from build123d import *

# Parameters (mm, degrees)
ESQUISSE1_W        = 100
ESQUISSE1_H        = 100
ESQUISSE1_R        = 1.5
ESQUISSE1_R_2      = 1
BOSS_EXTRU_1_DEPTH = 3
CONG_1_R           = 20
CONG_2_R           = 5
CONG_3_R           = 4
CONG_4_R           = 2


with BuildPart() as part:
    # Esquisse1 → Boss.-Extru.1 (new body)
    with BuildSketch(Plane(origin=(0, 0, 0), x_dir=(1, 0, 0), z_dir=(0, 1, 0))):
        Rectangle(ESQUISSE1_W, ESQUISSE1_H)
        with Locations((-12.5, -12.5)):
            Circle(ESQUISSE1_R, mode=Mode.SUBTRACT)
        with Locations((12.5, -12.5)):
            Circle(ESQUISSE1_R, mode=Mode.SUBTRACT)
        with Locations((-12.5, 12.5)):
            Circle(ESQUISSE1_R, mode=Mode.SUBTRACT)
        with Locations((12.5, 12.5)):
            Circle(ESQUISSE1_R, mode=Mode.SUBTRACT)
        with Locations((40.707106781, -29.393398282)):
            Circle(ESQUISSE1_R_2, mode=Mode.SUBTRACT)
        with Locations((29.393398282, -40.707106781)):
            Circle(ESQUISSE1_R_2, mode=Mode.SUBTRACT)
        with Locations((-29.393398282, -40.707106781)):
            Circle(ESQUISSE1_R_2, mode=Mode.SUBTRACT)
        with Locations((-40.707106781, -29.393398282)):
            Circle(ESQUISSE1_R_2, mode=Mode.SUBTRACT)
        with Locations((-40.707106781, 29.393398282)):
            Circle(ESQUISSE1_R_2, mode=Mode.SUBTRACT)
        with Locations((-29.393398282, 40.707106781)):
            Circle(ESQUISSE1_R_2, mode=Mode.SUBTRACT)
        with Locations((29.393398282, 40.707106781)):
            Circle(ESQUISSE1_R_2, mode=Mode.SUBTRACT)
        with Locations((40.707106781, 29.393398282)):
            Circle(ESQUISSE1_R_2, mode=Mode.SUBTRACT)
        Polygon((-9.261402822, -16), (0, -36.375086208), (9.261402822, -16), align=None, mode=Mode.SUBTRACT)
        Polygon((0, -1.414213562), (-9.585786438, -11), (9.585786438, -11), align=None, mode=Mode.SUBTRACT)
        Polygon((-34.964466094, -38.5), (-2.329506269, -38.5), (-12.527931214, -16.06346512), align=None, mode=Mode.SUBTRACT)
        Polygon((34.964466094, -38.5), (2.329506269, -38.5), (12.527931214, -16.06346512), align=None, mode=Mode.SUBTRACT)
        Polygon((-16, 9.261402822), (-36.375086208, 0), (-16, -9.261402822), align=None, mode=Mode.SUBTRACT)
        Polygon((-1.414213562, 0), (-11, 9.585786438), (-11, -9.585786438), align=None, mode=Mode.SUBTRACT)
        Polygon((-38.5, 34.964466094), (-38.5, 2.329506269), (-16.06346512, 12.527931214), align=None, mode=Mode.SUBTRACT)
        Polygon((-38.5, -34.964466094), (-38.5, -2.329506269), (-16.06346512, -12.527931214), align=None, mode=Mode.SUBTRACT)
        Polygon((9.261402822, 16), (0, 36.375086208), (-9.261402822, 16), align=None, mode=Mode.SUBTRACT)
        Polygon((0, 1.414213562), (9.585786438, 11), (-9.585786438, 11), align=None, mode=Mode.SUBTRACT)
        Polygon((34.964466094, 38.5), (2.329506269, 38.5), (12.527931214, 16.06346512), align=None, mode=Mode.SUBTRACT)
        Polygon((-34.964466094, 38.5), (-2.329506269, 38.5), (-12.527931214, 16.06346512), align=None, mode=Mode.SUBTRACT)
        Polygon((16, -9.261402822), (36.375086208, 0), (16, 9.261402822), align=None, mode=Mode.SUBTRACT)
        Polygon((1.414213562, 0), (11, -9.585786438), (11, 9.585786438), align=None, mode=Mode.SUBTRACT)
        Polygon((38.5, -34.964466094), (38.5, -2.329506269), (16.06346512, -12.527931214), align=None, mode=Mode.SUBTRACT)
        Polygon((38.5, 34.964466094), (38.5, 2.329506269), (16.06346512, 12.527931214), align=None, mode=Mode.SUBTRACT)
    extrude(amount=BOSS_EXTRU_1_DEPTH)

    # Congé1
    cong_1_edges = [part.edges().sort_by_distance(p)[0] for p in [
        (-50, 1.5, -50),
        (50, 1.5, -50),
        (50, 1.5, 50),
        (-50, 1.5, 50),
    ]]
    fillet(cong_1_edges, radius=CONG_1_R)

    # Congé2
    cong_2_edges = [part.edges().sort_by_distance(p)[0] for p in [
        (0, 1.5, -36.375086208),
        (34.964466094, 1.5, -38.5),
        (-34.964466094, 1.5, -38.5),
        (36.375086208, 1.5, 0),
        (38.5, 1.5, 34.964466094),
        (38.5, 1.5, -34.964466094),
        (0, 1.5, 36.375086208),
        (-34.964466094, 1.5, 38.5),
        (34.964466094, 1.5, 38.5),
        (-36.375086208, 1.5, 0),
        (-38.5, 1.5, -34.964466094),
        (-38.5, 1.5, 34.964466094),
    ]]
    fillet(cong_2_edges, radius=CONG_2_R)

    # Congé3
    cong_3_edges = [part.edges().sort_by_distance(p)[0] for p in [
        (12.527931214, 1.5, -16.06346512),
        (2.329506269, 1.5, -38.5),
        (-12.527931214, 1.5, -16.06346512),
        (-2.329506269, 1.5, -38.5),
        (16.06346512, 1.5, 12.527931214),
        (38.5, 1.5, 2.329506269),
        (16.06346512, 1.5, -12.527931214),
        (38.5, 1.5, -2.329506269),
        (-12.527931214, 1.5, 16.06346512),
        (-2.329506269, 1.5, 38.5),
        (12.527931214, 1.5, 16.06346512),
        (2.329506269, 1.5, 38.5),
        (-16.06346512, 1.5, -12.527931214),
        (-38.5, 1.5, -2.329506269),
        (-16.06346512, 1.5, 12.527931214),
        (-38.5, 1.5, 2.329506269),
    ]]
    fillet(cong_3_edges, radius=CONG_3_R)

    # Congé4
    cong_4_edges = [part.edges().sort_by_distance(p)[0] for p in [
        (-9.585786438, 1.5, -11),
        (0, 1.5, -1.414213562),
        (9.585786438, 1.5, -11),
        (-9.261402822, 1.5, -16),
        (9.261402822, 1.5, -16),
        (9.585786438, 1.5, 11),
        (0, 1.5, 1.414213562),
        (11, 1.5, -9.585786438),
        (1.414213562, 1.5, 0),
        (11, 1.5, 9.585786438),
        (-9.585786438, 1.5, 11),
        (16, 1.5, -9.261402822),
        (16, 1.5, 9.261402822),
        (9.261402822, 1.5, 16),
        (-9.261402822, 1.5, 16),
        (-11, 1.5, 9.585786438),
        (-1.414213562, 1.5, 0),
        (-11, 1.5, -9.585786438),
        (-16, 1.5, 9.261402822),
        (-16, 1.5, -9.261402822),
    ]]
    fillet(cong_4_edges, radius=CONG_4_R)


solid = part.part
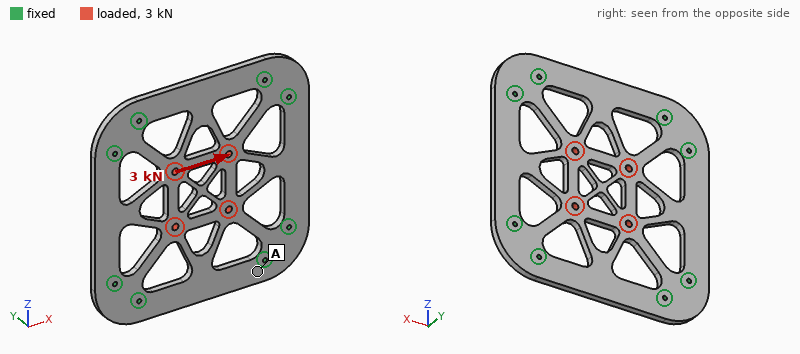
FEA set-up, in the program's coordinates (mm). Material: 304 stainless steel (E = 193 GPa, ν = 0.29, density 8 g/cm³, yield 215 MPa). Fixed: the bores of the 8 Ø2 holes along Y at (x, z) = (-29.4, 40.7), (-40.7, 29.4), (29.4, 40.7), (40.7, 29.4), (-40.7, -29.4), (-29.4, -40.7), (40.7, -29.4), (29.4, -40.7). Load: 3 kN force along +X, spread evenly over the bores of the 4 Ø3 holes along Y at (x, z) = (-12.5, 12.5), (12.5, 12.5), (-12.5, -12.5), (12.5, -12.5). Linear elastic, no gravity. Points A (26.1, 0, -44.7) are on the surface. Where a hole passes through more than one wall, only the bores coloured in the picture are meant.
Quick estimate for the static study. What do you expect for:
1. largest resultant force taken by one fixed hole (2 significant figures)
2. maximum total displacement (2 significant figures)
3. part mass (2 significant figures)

540 N
9.1 µm
150 g
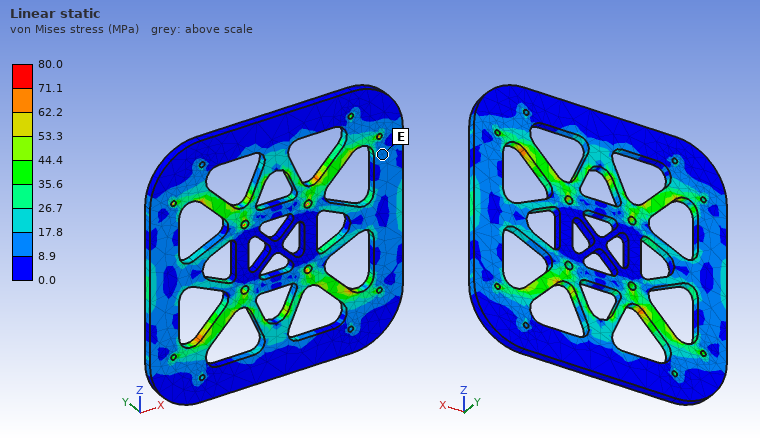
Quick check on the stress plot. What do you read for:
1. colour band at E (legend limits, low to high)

8.9 to 17.8 MPa
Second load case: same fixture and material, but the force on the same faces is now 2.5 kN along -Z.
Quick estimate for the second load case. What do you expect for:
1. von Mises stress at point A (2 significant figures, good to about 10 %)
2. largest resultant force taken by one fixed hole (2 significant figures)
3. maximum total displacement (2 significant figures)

6.1 MPa
450 N
7.6 µm
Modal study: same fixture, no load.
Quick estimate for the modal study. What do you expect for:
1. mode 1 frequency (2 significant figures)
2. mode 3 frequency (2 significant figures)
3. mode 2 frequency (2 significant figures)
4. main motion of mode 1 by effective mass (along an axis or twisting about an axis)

2000 Hz
3600 Hz
3600 Hz
along Y
